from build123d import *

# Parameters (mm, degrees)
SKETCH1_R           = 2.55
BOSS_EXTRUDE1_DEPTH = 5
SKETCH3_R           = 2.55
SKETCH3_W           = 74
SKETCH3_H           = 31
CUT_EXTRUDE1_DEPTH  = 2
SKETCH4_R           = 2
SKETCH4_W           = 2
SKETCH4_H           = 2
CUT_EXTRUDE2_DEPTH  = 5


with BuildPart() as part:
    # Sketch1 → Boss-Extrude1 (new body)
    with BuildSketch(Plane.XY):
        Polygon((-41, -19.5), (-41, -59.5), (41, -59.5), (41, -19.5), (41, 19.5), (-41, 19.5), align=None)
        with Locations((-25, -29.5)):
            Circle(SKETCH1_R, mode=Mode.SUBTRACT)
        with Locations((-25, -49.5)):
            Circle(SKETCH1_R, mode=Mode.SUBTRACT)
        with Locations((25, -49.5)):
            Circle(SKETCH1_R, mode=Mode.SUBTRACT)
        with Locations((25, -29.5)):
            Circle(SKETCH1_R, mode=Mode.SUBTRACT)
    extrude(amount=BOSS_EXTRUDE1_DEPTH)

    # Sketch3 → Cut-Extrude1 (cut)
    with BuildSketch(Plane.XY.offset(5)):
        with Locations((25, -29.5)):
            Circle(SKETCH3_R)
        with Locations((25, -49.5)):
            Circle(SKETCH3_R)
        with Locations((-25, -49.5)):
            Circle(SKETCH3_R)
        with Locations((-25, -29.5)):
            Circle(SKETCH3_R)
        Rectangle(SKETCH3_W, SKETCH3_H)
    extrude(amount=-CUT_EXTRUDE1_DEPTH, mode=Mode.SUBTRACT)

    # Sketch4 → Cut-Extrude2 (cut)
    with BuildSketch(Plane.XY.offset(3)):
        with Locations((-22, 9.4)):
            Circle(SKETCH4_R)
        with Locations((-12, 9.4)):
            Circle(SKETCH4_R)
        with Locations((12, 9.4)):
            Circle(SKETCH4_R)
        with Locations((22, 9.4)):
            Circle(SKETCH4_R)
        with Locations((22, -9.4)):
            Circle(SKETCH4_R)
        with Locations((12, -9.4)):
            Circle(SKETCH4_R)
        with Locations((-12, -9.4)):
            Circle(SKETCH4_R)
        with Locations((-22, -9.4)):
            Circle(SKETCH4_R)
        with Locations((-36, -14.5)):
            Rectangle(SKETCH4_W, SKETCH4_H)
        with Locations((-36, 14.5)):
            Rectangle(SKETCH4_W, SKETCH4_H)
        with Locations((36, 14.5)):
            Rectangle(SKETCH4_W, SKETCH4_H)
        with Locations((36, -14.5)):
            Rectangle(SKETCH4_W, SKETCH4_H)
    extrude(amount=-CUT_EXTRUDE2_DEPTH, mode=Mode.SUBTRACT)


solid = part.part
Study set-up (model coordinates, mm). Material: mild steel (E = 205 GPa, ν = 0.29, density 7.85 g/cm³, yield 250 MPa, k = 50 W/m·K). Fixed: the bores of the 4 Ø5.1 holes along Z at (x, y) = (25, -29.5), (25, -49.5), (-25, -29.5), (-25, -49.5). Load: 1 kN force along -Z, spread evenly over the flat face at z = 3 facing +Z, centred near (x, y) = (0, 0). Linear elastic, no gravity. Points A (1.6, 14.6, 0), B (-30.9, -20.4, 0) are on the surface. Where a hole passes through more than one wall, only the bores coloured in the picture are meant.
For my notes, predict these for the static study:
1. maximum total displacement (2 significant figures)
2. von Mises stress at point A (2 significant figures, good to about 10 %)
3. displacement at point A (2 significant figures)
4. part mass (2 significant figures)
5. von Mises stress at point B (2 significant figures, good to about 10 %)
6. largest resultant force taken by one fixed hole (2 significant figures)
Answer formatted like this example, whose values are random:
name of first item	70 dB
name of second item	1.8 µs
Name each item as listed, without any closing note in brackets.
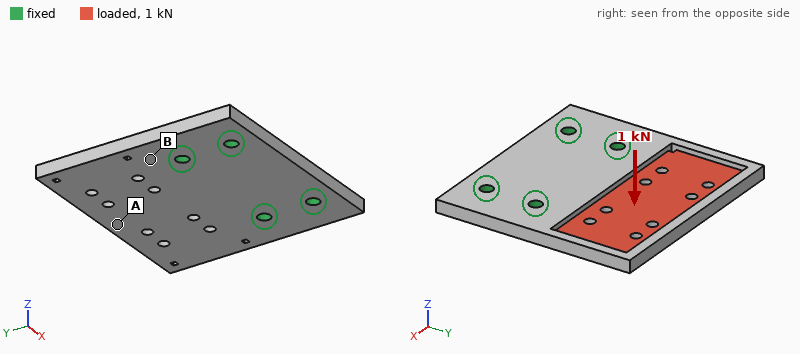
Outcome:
maximum total displacement	0.20 mm
von Mises stress at point A	17 MPa
displacement at point A	0.17 mm
part mass	210 g
von Mises stress at point B	65 MPa
largest resultant force taken by one fixed hole	790 N
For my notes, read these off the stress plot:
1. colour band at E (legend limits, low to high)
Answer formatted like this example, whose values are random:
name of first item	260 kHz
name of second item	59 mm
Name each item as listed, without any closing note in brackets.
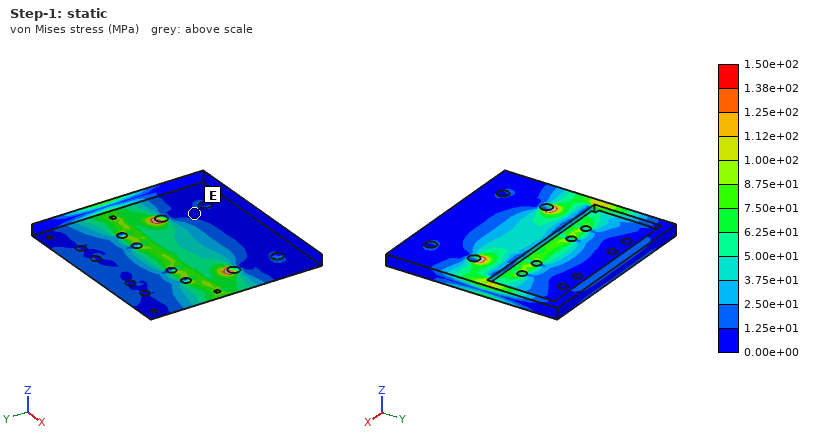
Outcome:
colour band at E	0.00e+00 to 1.25e+01 MPa
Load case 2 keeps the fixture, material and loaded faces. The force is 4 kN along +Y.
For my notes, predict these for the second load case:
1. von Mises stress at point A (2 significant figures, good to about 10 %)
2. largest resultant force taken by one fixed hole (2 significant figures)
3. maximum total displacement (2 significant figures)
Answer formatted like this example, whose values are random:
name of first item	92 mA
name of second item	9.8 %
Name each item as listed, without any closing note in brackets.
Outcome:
von Mises stress at point A	6.9 MPa
largest resultant force taken by one fixed hole	1.5 kN
maximum total displacement	60 µm
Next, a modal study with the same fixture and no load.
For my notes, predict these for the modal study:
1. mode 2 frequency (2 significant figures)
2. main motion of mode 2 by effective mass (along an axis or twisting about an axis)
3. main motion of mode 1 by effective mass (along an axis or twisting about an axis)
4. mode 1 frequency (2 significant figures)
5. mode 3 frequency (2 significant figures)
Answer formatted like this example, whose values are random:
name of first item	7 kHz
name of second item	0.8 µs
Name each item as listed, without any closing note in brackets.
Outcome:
mode 2 frequency	2200 Hz
main motion of mode 2 by effective mass	twisting about Y
main motion of mode 1 by effective mass	along Z
mode 1 frequency	1500 Hz
mode 3 frequency	4500 Hz
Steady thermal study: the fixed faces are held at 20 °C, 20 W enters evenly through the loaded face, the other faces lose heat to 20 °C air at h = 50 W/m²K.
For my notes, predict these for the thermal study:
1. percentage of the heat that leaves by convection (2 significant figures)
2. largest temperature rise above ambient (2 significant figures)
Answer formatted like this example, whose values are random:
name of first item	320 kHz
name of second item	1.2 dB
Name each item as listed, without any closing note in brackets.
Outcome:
percentage of the heat that leaves by convection	37 %
largest temperature rise above ambient	31 K
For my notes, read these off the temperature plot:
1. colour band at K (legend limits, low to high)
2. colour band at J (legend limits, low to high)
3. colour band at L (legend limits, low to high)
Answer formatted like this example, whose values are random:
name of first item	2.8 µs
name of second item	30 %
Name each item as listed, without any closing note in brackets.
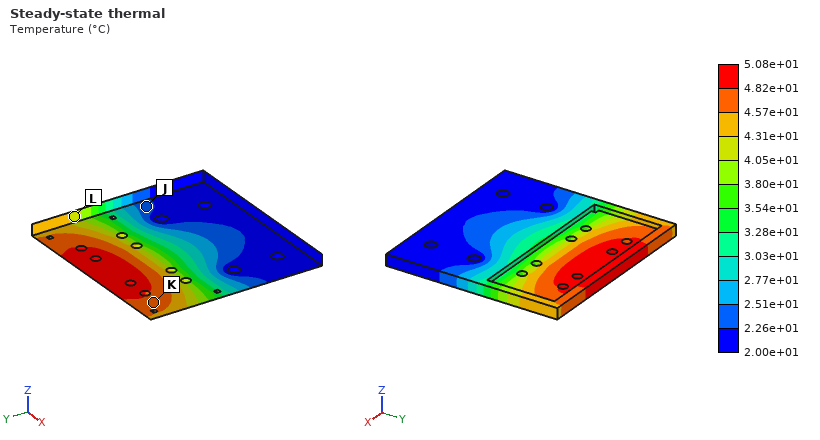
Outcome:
colour band at K	4.57e+01 to 4.82e+01 °C
colour band at J	2.26e+01 to 2.51e+01 °C
colour band at L	4.05e+01 to 4.31e+01 °C
